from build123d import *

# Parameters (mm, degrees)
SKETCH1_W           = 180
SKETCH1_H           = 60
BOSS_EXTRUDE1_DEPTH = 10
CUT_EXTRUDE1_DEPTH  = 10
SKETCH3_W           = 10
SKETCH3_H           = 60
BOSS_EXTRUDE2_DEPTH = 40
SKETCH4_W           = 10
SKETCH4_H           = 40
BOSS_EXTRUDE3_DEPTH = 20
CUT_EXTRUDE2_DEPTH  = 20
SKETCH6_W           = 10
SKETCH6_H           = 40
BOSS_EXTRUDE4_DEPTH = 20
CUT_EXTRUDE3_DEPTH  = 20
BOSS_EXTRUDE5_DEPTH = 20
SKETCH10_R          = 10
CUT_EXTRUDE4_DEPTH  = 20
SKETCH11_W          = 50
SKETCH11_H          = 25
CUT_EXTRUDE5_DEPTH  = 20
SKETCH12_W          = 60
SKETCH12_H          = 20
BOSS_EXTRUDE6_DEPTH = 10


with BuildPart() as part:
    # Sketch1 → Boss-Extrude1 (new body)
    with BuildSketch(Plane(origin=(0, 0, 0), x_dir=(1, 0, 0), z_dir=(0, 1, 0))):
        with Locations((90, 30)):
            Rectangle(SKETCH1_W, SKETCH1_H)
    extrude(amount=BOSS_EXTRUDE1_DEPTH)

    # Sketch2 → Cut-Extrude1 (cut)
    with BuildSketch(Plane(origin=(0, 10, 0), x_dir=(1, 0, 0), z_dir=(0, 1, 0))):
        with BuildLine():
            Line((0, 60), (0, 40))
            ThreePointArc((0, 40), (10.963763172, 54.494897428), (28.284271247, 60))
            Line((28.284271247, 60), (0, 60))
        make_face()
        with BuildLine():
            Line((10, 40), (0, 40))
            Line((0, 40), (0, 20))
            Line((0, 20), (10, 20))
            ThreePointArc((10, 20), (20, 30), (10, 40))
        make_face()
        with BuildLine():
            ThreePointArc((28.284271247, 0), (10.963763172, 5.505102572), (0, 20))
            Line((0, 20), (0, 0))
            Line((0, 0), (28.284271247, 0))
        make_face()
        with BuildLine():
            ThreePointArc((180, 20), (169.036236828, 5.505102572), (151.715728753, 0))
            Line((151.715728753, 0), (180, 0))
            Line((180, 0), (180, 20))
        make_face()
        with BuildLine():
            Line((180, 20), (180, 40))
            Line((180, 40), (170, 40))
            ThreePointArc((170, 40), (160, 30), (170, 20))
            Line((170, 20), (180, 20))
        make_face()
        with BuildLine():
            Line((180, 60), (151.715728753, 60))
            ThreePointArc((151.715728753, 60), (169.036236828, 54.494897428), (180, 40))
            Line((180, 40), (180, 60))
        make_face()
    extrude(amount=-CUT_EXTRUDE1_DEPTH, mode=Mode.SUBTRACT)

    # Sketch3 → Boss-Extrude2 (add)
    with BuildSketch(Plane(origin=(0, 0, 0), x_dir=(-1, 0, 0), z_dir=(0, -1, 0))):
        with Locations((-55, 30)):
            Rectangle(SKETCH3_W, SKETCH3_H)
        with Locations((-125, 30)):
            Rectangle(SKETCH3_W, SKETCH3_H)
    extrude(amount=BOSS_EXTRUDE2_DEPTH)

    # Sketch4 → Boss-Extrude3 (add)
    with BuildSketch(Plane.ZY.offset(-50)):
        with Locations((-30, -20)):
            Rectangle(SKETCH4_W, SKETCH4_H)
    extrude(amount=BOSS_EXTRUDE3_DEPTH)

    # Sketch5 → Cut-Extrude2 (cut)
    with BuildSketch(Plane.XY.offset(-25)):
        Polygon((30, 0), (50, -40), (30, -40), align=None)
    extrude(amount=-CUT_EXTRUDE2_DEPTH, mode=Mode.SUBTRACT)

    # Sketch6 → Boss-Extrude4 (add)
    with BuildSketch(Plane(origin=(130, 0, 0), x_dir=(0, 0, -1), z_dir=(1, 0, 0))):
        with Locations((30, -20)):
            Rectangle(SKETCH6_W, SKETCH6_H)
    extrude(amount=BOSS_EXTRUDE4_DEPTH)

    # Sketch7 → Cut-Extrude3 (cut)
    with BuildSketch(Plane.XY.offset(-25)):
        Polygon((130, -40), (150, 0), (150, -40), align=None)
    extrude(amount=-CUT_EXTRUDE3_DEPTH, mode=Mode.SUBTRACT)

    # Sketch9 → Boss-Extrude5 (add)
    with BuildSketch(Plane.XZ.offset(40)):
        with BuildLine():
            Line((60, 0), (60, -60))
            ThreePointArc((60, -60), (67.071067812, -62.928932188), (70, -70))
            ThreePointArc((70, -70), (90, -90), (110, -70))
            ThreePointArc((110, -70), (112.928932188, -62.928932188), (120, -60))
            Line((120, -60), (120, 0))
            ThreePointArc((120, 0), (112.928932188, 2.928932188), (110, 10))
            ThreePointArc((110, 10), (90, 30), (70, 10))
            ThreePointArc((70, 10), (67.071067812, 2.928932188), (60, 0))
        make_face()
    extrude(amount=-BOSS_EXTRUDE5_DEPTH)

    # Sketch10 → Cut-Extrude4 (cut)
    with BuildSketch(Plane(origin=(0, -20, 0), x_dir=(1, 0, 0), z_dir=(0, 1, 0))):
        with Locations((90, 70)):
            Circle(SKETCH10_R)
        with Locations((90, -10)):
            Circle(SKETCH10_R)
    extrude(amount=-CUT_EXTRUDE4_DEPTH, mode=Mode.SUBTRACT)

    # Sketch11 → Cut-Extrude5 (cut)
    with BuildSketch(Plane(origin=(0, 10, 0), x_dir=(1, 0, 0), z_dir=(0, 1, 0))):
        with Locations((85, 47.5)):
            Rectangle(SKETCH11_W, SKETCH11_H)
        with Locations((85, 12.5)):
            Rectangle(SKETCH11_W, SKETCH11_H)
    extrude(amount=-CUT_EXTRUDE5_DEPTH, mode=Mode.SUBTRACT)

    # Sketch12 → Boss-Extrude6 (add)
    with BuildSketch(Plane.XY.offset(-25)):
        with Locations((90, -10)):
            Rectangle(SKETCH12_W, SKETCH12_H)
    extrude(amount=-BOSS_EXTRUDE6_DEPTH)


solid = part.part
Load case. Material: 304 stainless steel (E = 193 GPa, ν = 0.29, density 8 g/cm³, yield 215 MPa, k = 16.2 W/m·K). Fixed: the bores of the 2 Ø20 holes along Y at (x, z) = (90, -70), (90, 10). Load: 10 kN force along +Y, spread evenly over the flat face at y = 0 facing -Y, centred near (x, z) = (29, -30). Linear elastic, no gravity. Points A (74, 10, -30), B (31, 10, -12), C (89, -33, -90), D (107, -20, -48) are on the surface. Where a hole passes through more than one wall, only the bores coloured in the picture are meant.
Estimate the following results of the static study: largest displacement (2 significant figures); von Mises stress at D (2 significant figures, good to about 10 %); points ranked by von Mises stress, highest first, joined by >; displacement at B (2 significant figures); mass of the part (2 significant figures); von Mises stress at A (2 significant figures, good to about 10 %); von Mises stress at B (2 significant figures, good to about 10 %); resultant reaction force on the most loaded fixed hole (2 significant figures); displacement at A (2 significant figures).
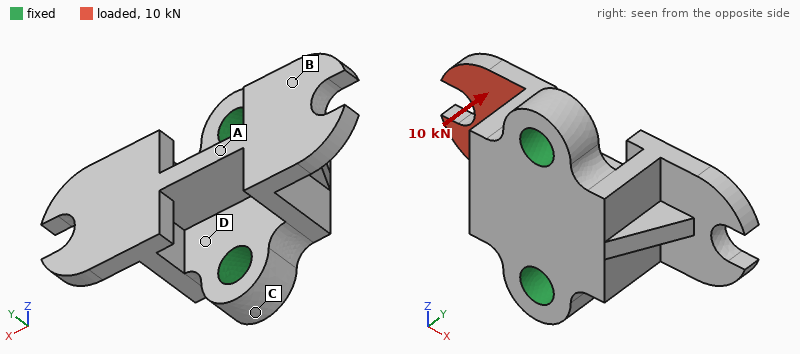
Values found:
0.18 mm
24 MPa
A > B > D > C
0.094 mm
1.9 kg
61 MPa
45 MPa
5.4 kN
0.035 mm
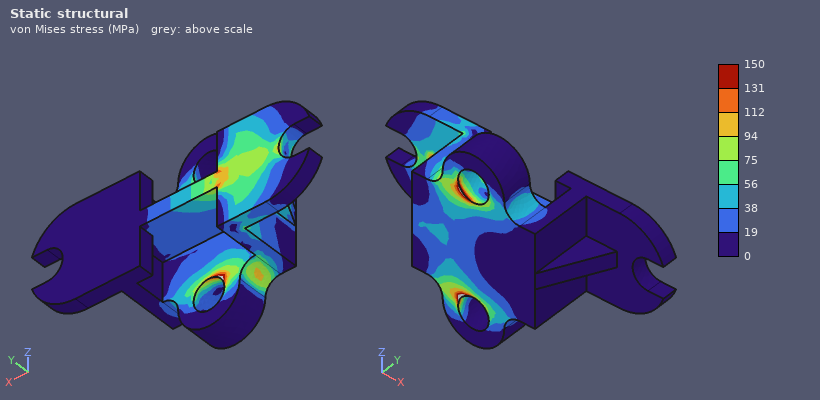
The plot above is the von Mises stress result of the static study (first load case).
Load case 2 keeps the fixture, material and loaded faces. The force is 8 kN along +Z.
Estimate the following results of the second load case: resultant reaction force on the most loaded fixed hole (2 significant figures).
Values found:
8.2 kN
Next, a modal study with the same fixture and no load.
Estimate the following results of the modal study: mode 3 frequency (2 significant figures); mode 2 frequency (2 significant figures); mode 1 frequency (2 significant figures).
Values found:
4000 Hz
3900 Hz
2500 Hz
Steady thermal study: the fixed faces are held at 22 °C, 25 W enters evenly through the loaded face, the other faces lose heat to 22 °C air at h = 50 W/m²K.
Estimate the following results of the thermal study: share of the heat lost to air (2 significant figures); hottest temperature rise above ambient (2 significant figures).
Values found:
77 %
59 K
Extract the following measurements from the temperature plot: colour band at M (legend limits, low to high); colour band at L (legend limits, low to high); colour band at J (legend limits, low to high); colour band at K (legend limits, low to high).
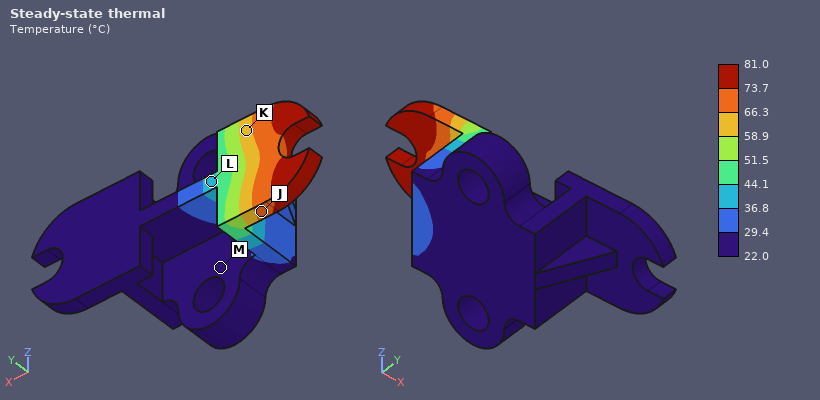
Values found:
22.0 to 29.4 °C
36.8 to 44.1 °C
66.3 to 73.7 °C
58.9 to 66.3 °C
